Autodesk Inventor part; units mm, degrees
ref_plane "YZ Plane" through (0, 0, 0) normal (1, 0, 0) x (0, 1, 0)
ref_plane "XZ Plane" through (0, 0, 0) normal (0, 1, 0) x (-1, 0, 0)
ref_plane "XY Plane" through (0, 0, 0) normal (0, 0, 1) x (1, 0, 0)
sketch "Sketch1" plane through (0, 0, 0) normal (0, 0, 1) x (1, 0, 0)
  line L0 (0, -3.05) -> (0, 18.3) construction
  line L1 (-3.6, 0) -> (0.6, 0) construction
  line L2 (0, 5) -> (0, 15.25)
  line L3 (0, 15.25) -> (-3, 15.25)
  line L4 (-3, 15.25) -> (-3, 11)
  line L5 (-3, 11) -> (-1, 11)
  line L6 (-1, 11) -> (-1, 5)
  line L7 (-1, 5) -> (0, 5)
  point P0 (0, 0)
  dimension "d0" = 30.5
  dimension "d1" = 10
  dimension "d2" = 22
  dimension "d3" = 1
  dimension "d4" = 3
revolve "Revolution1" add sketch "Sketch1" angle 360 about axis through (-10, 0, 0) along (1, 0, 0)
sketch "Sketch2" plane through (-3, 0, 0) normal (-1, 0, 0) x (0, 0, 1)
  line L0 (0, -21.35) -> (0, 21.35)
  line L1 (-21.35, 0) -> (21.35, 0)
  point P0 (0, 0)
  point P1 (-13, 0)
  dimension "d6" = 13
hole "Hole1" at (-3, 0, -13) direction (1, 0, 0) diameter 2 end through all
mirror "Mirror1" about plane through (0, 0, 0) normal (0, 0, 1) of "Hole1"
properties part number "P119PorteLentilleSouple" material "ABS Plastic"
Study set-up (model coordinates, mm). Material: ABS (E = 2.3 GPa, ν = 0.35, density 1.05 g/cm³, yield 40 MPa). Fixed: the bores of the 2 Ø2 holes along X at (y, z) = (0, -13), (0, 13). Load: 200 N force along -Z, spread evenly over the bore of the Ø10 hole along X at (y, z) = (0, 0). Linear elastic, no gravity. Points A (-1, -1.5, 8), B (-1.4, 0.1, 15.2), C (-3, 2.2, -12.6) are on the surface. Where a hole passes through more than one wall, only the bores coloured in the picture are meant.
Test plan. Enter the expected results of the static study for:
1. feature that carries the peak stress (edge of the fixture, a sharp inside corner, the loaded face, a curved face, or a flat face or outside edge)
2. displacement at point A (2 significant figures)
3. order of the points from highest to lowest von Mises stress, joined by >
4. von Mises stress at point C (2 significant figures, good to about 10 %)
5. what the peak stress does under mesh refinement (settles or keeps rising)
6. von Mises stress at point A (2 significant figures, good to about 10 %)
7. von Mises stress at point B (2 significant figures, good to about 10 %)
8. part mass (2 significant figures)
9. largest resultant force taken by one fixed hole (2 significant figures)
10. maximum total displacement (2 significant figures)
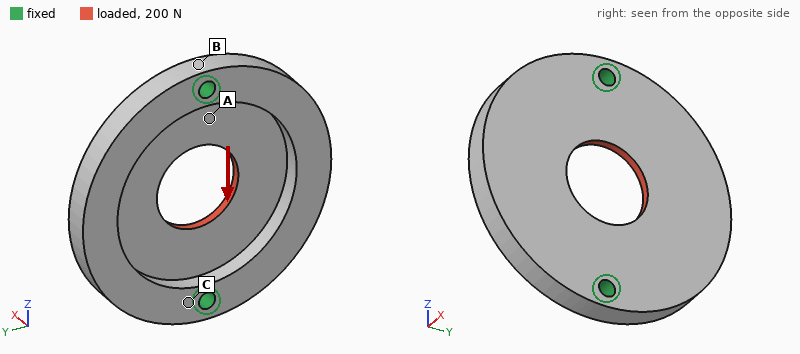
edge of the fixture
26 µm
A > B > C
2.7 MPa
keeps rising
11 MPa
7.8 MPa
1.4 g
100 N
53 µm
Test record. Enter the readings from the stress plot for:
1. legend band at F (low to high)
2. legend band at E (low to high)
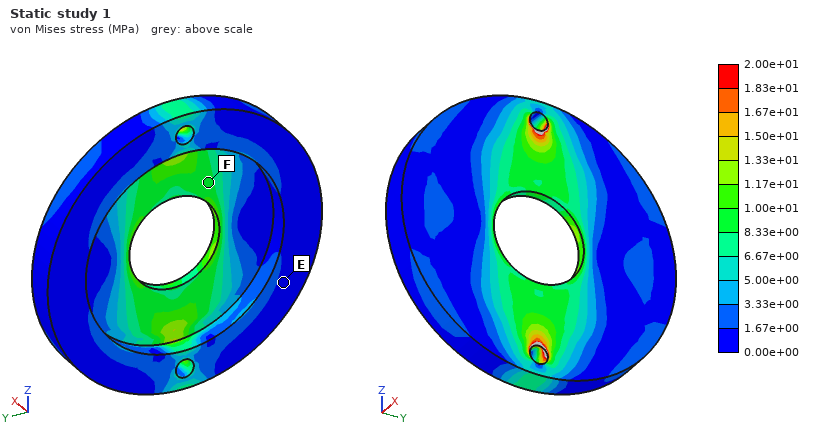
8.33e+00 to 1.00e+01 MPa
0.00e+00 to 1.67e+00 MPa
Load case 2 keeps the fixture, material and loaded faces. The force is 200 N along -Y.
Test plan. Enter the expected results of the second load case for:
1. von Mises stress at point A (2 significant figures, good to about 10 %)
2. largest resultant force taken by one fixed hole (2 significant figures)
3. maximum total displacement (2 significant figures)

8.0 MPa
100 N
0.16 mm
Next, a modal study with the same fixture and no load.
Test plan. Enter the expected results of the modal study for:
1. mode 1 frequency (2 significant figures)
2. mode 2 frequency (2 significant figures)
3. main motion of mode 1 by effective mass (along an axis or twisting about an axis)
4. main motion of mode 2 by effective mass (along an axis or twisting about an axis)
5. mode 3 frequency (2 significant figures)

2200 Hz
2400 Hz
twisting about Z
along X
5900 Hz
